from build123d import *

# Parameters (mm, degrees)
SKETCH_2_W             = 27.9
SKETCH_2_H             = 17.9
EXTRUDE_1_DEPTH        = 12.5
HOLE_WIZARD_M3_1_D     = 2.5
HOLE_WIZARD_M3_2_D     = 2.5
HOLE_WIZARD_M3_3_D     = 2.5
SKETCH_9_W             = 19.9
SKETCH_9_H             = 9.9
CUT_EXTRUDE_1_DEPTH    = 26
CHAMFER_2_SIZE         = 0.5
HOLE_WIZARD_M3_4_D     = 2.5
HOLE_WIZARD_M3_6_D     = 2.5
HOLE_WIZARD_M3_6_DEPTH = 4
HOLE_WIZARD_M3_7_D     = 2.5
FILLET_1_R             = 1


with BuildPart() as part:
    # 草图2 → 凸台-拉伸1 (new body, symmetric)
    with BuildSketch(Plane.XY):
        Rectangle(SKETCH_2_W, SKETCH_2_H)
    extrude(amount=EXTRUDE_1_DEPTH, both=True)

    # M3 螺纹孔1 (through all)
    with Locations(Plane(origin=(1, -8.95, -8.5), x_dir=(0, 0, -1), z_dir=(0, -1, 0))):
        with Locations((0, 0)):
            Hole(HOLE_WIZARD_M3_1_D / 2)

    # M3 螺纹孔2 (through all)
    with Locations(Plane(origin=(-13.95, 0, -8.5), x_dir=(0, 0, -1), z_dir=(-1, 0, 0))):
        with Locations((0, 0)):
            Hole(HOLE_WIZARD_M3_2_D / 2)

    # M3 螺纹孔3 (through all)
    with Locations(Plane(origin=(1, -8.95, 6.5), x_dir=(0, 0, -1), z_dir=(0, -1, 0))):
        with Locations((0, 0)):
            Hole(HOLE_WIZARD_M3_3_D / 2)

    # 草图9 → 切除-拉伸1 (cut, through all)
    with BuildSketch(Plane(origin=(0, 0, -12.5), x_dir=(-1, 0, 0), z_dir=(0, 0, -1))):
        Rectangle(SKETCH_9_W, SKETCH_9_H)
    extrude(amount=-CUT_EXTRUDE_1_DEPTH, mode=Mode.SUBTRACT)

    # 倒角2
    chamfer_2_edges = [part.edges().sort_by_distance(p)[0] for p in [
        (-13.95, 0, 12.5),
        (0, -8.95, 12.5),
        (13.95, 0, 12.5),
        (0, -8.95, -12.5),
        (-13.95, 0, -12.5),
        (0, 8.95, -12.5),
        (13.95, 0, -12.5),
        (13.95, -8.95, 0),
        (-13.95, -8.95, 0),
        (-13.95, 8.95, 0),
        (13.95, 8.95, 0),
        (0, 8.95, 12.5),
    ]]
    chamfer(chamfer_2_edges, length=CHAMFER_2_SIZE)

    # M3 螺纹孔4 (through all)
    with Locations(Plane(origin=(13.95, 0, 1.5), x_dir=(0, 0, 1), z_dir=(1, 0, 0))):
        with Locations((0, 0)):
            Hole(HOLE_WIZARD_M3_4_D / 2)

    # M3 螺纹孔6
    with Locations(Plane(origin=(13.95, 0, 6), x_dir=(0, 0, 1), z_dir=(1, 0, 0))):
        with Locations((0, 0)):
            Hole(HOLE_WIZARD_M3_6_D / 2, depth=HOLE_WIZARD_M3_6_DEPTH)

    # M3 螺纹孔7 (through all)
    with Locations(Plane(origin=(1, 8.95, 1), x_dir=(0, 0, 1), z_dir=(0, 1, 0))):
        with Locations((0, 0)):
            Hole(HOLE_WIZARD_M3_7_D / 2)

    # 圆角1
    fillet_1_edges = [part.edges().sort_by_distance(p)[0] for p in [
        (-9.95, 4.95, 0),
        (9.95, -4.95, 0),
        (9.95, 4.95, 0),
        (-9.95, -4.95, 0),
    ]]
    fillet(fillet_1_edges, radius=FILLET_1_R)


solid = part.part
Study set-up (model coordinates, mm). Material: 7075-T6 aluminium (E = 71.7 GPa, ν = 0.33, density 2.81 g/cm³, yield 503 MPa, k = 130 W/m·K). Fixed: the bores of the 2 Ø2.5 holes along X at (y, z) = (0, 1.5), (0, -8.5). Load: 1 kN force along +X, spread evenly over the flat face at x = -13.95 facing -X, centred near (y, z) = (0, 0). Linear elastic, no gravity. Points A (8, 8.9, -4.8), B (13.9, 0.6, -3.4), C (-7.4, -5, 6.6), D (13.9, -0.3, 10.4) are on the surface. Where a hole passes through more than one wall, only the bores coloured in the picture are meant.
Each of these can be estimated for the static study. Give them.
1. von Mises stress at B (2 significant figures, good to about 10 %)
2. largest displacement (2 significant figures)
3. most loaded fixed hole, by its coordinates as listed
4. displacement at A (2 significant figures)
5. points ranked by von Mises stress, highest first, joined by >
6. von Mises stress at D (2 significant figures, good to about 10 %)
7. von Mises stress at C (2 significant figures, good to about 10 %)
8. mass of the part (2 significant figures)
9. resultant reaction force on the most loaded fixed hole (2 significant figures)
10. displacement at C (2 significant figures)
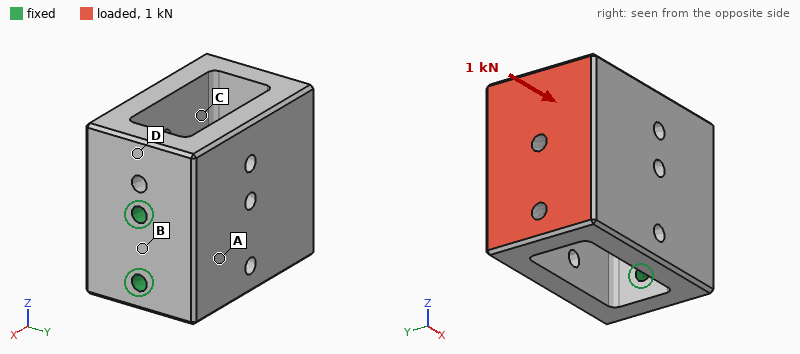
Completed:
27 MPa
16 µm
(0, 1.5)
6.0 µm
B > D > C > A
18 MPa
9.8 MPa
21 g
760 N
12 µm
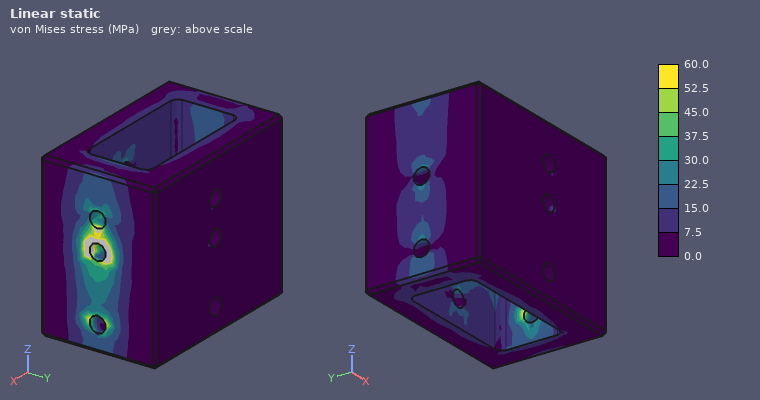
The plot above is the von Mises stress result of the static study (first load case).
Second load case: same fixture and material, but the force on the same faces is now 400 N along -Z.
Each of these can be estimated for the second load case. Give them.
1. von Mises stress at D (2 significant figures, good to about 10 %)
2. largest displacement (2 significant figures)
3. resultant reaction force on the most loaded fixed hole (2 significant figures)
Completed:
16 MPa
39 µm
800 N
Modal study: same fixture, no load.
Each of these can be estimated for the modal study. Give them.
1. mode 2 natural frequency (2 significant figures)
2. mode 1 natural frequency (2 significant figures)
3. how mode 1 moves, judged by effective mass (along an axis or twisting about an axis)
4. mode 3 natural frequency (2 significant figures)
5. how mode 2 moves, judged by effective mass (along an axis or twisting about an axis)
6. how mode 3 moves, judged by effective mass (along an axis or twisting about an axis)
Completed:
6000 Hz
3500 Hz
along Y
11 kHz
along Z
twisting about X
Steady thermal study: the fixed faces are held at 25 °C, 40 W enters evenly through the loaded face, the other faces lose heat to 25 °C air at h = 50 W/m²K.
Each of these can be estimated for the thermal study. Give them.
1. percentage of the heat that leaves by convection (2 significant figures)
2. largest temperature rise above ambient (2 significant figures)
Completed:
13 %
49 K
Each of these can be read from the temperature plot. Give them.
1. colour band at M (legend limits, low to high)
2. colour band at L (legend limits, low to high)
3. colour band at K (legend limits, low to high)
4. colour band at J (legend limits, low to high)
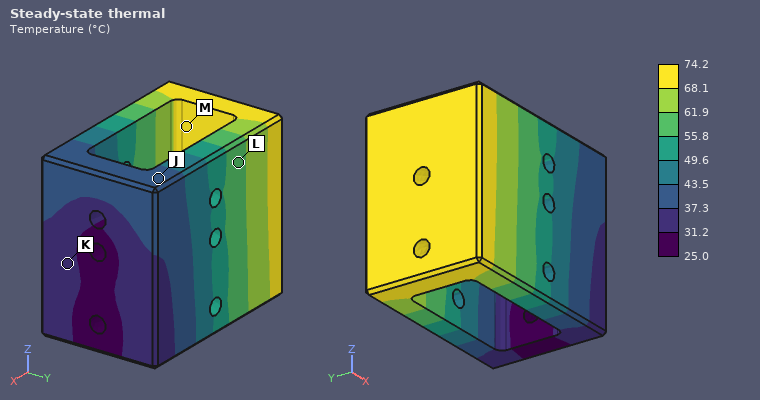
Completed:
68.1 to 74.2 °C
55.8 to 61.9 °C
31.2 to 37.3 °C
37.3 to 43.5 °C
